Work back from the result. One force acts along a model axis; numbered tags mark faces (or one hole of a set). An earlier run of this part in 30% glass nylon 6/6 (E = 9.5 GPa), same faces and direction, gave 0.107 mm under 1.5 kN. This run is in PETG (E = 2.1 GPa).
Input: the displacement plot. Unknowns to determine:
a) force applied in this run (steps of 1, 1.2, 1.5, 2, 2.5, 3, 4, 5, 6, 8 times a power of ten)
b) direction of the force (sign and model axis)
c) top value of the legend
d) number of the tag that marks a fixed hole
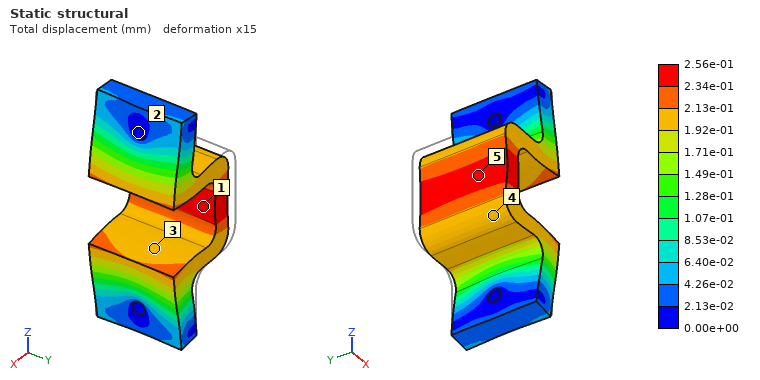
800 N
+X
2.56e-01 mm
2
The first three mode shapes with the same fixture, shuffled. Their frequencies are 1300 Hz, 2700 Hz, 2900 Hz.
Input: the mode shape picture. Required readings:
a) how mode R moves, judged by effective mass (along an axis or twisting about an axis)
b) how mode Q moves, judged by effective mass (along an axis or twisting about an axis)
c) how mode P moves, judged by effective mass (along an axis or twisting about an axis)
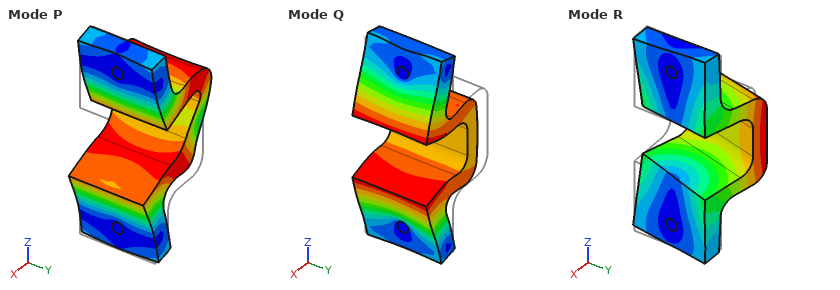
along Y
along X
along Z
